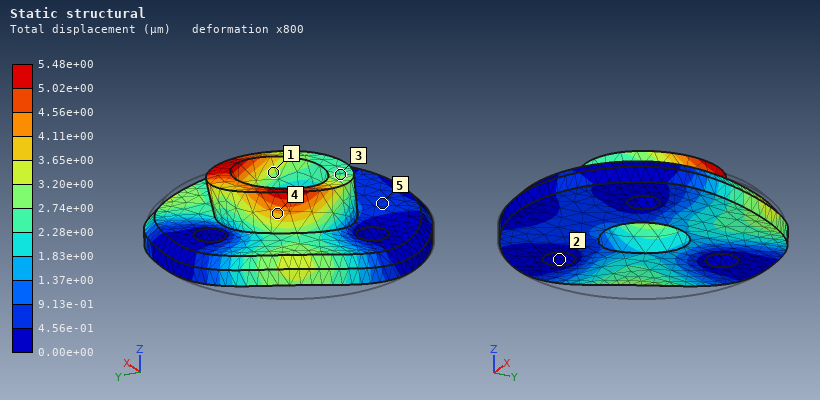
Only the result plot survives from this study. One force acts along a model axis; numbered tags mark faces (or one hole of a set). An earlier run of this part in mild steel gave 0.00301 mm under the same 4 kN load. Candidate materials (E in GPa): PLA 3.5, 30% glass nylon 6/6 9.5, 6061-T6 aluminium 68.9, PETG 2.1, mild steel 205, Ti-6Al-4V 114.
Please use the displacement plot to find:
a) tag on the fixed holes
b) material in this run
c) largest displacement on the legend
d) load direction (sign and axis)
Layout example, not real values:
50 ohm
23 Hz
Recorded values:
2
Ti-6Al-4V
5.48e+00 µm
+X
